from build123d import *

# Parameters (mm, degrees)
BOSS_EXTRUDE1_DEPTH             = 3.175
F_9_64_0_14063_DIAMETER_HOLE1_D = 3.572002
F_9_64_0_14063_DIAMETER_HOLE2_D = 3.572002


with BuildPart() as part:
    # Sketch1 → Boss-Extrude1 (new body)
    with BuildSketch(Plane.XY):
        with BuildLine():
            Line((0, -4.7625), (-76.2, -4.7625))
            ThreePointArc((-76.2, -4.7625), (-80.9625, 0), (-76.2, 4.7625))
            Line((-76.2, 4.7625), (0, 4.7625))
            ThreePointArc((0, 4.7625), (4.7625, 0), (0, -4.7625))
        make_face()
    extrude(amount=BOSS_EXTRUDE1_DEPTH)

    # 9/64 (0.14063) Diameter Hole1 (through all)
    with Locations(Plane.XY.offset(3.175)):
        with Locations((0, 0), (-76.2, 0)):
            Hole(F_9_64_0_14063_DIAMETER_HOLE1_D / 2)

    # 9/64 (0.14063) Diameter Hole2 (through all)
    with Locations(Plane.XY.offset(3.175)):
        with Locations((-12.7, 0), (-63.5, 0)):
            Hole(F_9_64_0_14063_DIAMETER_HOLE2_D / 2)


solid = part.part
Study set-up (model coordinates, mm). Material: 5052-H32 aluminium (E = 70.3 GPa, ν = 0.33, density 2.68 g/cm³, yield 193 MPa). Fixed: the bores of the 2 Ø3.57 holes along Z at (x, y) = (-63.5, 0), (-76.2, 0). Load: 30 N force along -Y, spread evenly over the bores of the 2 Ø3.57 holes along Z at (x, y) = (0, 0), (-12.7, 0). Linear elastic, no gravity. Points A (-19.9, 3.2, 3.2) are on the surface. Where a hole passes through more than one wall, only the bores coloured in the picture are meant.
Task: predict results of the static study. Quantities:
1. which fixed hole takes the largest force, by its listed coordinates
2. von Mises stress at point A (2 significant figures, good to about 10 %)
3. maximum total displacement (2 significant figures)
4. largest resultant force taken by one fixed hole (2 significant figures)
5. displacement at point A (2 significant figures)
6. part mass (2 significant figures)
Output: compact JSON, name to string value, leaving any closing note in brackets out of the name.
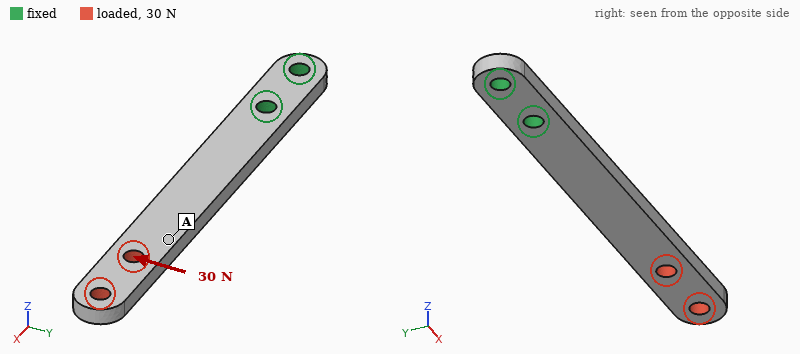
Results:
{"which fixed hole takes the largest force, by its listed coordinates": "(-63.5, 0)", "von Mises stress at point A": "5.8 MPa", "maximum total displacement": "0.17 mm", "largest resultant force taken by one fixed hole": "82 N", "displacement at point A": "0.087 mm", "part mass": "6.4 g"}
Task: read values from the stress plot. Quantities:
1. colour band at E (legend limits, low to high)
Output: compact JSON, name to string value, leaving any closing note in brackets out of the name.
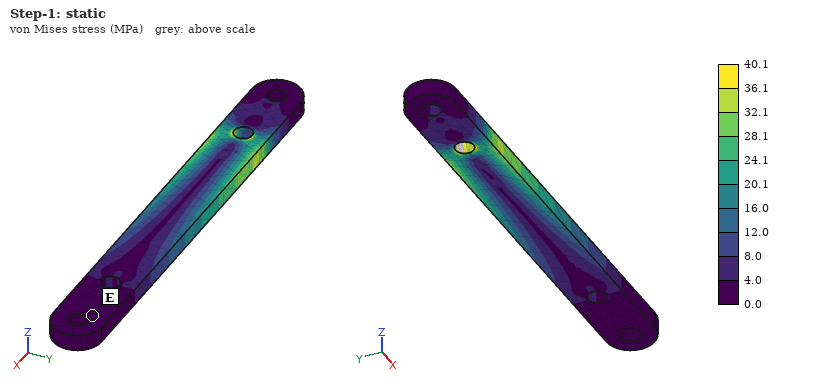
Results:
{"colour band at E": "0.0 to 4.0 MPa"}
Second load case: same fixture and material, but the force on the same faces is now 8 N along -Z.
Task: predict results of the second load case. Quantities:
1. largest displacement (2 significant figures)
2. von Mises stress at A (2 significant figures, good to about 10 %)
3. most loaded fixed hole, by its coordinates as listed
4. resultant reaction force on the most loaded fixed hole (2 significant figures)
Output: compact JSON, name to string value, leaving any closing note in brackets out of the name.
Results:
{"largest displacement": "0.35 mm", "von Mises stress at A": "6.8 MPa", "most loaded fixed hole, by its coordinates as listed": "(-63.5, 0)", "resultant reaction force on the most loaded fixed hole": "10 N"}
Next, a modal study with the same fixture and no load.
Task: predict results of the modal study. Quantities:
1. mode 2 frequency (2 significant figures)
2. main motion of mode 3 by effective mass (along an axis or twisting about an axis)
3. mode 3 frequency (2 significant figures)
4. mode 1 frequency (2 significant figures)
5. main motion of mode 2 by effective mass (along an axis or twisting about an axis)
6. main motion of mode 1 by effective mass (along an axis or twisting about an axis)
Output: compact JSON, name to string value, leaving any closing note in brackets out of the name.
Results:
{"mode 2 frequency": "1700 Hz", "main motion of mode 3 by effective mass": "along Z", "mode 3 frequency": "3700 Hz", "mode 1 frequency": "620 Hz", "main motion of mode 2 by effective mass": "along Y", "main motion of mode 1 by effective mass": "along Z"}
